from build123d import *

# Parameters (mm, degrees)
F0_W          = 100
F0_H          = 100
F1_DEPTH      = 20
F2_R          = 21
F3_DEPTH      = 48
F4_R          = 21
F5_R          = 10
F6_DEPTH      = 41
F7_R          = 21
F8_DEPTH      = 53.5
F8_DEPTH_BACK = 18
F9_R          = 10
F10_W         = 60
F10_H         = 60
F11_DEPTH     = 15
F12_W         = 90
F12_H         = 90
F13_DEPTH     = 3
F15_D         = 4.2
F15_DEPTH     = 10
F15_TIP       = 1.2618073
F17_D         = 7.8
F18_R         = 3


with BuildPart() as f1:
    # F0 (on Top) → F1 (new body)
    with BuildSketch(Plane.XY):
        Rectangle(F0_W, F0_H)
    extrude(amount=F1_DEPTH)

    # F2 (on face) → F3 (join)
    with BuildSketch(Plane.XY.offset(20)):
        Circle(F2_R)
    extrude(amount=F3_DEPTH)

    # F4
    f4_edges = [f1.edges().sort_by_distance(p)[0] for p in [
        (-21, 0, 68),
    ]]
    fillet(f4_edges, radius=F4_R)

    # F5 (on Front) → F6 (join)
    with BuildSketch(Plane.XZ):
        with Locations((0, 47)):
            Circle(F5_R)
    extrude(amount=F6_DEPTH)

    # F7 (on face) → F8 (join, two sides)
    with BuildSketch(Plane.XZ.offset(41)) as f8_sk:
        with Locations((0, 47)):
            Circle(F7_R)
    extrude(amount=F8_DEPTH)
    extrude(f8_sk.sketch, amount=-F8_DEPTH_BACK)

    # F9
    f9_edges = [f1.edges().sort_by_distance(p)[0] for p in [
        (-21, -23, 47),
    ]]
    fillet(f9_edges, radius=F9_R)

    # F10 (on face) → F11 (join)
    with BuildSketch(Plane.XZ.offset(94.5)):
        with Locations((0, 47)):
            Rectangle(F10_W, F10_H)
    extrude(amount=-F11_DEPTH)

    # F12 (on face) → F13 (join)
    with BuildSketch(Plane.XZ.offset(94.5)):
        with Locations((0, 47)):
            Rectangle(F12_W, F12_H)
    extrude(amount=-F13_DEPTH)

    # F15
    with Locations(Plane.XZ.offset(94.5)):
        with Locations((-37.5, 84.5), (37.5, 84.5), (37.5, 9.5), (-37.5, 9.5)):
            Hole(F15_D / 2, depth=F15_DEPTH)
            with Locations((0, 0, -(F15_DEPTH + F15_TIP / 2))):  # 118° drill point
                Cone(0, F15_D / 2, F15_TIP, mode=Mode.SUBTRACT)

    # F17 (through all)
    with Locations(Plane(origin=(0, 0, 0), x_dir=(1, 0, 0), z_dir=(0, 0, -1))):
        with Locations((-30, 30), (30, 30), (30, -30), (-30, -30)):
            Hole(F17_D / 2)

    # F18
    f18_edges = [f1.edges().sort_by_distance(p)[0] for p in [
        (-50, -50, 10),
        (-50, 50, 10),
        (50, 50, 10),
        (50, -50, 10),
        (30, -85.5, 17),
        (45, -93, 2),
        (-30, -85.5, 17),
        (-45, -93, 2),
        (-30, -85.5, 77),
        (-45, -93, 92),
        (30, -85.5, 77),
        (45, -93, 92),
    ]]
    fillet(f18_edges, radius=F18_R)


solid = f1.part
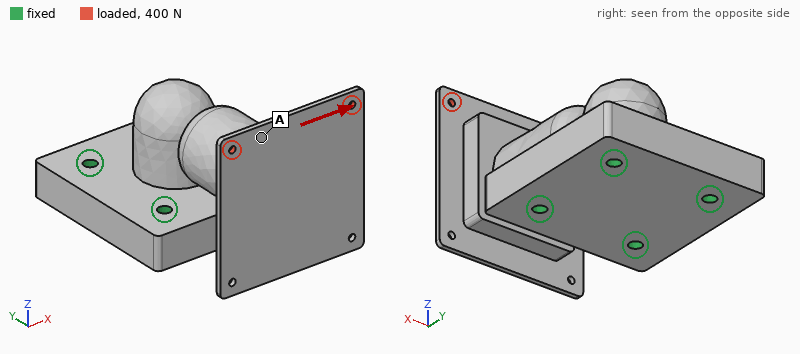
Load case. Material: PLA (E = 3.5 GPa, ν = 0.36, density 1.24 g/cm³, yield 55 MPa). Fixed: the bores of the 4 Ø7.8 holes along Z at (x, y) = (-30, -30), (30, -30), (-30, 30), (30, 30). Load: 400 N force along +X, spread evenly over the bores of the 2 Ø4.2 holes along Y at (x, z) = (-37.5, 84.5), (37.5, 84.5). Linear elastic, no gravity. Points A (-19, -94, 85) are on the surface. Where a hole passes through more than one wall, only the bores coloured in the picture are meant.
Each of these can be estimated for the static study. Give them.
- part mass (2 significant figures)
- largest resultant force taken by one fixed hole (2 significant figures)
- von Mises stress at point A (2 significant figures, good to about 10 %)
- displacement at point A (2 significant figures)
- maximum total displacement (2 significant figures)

490 g
360 N
3.0 MPa
1.9 mm
2.1 mm
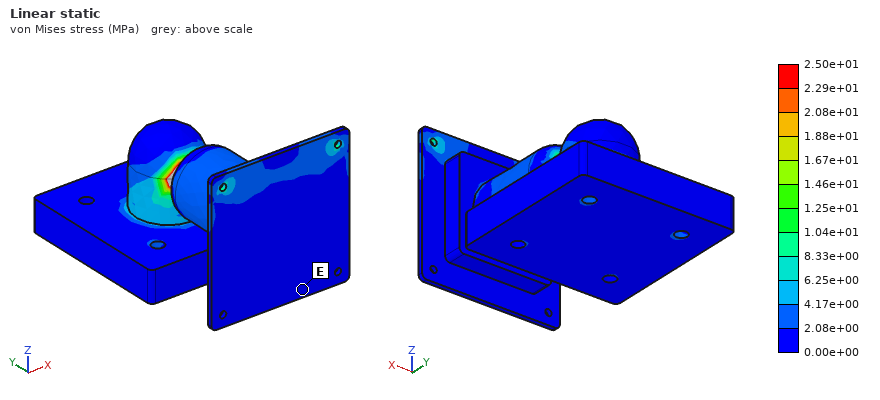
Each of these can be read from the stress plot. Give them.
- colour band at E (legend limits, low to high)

0.00e+00 to 2.08e+00 MPa
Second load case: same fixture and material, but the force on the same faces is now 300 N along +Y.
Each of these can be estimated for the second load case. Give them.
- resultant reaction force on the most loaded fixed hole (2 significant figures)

210 N
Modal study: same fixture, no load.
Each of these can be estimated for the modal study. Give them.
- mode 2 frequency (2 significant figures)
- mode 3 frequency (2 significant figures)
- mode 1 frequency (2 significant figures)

280 Hz
630 Hz
270 Hz
